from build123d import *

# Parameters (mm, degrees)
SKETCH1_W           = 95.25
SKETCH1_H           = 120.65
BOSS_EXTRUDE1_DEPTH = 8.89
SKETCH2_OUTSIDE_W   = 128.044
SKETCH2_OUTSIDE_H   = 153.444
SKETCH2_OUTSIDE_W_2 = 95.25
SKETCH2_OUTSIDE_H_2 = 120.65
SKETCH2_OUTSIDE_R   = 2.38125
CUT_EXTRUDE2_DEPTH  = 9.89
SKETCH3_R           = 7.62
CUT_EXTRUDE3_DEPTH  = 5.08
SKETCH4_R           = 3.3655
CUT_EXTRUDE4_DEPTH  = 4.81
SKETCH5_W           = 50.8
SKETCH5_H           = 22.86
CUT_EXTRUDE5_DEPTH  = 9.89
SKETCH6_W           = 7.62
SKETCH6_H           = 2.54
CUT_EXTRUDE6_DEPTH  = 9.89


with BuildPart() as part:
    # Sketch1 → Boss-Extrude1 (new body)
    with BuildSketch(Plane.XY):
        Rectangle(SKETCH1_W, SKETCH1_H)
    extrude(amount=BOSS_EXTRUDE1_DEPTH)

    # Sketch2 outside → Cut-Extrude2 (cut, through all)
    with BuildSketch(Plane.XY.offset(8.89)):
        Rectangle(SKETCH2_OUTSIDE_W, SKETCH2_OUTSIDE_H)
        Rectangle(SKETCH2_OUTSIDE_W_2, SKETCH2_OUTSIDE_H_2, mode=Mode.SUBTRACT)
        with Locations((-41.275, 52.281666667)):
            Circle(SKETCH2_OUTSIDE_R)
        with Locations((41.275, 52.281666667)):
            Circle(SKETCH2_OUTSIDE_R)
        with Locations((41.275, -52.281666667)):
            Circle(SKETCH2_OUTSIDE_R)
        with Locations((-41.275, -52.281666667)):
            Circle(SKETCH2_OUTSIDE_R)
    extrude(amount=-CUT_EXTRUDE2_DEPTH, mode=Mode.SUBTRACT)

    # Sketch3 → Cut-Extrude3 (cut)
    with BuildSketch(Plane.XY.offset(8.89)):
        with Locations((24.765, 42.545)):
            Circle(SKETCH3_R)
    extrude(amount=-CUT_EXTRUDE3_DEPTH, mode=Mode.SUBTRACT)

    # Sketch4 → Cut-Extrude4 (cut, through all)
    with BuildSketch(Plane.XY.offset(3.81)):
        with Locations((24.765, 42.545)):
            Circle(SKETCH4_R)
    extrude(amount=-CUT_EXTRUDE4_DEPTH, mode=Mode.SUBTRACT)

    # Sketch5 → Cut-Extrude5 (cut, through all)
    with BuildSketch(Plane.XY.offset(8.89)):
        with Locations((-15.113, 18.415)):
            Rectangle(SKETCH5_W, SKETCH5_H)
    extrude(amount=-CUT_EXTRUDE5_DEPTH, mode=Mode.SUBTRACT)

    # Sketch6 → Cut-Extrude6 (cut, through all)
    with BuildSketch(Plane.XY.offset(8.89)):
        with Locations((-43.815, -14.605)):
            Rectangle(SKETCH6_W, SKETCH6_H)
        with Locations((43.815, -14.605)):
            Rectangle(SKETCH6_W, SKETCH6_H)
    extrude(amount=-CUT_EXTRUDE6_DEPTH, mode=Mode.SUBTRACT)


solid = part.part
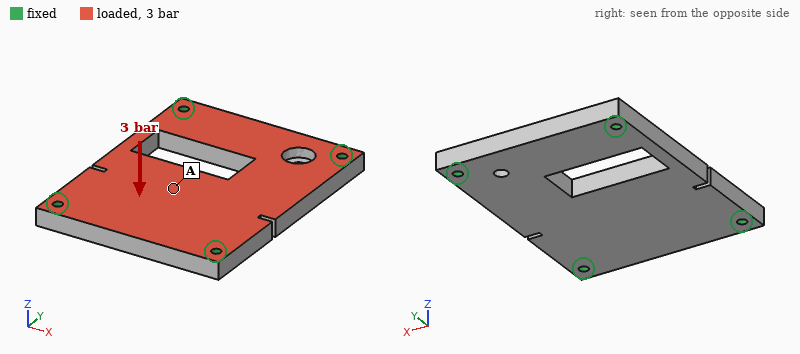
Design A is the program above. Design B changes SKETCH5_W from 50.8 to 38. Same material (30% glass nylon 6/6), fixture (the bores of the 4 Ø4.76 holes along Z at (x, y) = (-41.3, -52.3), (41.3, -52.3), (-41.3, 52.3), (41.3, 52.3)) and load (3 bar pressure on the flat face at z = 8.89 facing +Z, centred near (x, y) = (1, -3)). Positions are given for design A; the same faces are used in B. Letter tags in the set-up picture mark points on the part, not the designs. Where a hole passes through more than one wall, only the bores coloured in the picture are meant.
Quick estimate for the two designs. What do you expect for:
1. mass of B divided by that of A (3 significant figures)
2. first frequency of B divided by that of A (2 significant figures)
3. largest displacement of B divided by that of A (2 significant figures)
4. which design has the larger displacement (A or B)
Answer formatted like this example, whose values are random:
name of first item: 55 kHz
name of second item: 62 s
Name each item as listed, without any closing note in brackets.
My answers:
mass of B divided by that of A: 1.03
first frequency of B divided by that of A: 1.0
largest displacement of B divided by that of A: 0.90
which design has the larger displacement: A
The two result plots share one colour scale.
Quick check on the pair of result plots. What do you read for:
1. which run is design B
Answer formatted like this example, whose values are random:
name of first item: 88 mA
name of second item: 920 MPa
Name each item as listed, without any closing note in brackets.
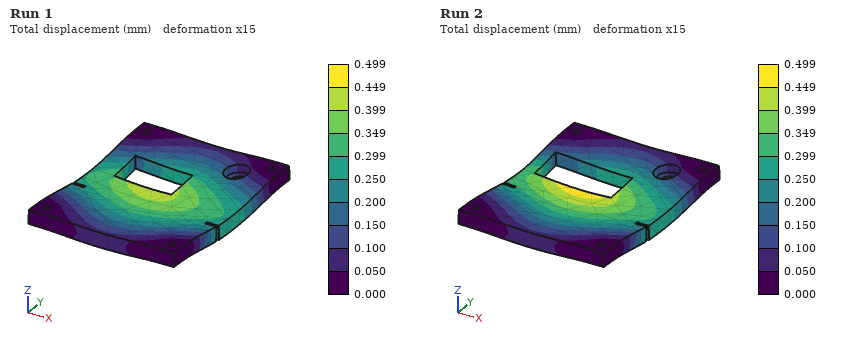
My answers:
which run is design B: Run 1
